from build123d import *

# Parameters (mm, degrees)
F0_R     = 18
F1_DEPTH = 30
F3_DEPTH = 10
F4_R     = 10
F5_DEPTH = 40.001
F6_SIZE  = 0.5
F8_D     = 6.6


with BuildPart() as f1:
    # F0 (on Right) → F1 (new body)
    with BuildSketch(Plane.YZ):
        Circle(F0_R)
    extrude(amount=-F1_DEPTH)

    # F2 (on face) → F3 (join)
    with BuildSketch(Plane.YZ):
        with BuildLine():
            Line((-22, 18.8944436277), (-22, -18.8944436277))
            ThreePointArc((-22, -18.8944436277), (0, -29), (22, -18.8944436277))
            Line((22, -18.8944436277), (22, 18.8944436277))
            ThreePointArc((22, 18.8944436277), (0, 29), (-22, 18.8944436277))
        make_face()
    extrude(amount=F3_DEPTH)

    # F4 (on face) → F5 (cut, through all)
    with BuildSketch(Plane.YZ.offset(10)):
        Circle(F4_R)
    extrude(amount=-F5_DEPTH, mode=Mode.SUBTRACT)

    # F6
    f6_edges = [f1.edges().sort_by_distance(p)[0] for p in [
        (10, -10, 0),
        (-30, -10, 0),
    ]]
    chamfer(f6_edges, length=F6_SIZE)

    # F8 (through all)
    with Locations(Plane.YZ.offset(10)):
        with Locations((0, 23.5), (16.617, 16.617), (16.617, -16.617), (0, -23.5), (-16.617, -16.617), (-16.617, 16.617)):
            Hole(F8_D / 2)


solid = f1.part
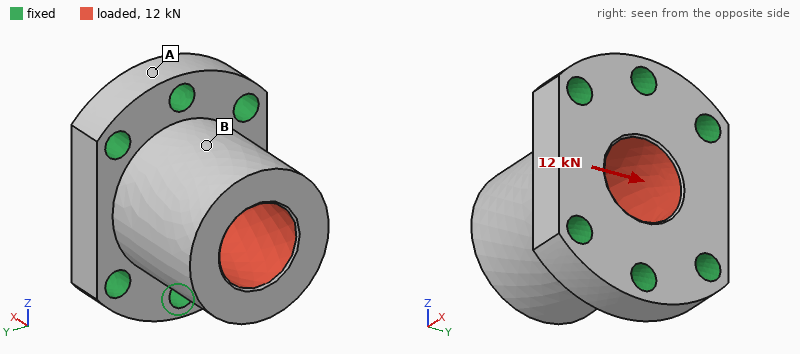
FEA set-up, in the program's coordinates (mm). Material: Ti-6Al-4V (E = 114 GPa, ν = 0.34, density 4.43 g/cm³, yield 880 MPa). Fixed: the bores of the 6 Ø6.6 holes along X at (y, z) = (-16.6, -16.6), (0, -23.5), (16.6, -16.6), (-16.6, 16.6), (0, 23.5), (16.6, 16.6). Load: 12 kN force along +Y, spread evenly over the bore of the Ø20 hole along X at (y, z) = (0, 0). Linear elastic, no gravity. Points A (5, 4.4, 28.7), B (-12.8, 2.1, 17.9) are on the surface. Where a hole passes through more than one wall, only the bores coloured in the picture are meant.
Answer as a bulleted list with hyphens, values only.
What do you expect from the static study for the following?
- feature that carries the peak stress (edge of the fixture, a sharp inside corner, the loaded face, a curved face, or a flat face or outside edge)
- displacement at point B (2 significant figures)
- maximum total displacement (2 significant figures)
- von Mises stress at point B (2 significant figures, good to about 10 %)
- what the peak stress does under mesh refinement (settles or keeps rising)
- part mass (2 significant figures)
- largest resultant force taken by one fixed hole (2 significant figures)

- edge of the fixture
- 11 µm
- 23 µm
- 17 MPa
- keeps rising
- 170 g
- 3.8 kN
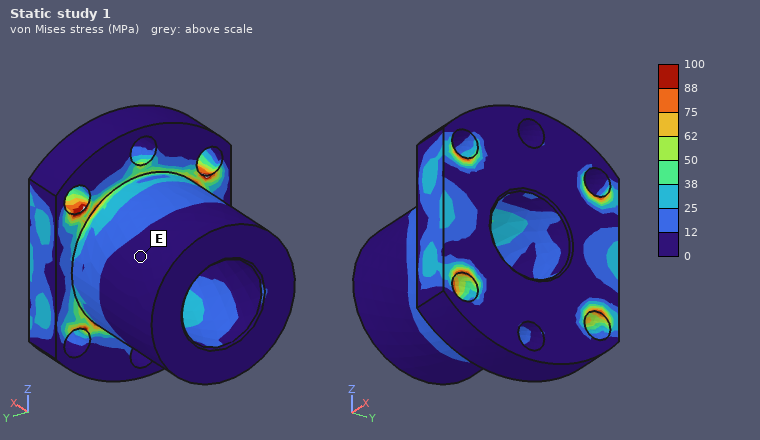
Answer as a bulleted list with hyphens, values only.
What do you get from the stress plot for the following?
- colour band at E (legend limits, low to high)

- 0 to 12 MPa
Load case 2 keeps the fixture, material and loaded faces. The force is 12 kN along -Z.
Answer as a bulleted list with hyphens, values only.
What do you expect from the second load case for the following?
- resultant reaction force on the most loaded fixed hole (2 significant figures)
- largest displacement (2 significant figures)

- 3.2 kN
- 17 µm
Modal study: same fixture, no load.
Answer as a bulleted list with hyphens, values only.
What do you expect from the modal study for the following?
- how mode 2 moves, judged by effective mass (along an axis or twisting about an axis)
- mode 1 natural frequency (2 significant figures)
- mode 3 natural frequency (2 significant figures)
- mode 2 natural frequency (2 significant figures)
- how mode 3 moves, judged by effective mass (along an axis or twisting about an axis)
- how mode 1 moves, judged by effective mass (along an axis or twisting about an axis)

- along Z
- 12 kHz
- 22 kHz
- 14 kHz
- twisting about X
- along Y
